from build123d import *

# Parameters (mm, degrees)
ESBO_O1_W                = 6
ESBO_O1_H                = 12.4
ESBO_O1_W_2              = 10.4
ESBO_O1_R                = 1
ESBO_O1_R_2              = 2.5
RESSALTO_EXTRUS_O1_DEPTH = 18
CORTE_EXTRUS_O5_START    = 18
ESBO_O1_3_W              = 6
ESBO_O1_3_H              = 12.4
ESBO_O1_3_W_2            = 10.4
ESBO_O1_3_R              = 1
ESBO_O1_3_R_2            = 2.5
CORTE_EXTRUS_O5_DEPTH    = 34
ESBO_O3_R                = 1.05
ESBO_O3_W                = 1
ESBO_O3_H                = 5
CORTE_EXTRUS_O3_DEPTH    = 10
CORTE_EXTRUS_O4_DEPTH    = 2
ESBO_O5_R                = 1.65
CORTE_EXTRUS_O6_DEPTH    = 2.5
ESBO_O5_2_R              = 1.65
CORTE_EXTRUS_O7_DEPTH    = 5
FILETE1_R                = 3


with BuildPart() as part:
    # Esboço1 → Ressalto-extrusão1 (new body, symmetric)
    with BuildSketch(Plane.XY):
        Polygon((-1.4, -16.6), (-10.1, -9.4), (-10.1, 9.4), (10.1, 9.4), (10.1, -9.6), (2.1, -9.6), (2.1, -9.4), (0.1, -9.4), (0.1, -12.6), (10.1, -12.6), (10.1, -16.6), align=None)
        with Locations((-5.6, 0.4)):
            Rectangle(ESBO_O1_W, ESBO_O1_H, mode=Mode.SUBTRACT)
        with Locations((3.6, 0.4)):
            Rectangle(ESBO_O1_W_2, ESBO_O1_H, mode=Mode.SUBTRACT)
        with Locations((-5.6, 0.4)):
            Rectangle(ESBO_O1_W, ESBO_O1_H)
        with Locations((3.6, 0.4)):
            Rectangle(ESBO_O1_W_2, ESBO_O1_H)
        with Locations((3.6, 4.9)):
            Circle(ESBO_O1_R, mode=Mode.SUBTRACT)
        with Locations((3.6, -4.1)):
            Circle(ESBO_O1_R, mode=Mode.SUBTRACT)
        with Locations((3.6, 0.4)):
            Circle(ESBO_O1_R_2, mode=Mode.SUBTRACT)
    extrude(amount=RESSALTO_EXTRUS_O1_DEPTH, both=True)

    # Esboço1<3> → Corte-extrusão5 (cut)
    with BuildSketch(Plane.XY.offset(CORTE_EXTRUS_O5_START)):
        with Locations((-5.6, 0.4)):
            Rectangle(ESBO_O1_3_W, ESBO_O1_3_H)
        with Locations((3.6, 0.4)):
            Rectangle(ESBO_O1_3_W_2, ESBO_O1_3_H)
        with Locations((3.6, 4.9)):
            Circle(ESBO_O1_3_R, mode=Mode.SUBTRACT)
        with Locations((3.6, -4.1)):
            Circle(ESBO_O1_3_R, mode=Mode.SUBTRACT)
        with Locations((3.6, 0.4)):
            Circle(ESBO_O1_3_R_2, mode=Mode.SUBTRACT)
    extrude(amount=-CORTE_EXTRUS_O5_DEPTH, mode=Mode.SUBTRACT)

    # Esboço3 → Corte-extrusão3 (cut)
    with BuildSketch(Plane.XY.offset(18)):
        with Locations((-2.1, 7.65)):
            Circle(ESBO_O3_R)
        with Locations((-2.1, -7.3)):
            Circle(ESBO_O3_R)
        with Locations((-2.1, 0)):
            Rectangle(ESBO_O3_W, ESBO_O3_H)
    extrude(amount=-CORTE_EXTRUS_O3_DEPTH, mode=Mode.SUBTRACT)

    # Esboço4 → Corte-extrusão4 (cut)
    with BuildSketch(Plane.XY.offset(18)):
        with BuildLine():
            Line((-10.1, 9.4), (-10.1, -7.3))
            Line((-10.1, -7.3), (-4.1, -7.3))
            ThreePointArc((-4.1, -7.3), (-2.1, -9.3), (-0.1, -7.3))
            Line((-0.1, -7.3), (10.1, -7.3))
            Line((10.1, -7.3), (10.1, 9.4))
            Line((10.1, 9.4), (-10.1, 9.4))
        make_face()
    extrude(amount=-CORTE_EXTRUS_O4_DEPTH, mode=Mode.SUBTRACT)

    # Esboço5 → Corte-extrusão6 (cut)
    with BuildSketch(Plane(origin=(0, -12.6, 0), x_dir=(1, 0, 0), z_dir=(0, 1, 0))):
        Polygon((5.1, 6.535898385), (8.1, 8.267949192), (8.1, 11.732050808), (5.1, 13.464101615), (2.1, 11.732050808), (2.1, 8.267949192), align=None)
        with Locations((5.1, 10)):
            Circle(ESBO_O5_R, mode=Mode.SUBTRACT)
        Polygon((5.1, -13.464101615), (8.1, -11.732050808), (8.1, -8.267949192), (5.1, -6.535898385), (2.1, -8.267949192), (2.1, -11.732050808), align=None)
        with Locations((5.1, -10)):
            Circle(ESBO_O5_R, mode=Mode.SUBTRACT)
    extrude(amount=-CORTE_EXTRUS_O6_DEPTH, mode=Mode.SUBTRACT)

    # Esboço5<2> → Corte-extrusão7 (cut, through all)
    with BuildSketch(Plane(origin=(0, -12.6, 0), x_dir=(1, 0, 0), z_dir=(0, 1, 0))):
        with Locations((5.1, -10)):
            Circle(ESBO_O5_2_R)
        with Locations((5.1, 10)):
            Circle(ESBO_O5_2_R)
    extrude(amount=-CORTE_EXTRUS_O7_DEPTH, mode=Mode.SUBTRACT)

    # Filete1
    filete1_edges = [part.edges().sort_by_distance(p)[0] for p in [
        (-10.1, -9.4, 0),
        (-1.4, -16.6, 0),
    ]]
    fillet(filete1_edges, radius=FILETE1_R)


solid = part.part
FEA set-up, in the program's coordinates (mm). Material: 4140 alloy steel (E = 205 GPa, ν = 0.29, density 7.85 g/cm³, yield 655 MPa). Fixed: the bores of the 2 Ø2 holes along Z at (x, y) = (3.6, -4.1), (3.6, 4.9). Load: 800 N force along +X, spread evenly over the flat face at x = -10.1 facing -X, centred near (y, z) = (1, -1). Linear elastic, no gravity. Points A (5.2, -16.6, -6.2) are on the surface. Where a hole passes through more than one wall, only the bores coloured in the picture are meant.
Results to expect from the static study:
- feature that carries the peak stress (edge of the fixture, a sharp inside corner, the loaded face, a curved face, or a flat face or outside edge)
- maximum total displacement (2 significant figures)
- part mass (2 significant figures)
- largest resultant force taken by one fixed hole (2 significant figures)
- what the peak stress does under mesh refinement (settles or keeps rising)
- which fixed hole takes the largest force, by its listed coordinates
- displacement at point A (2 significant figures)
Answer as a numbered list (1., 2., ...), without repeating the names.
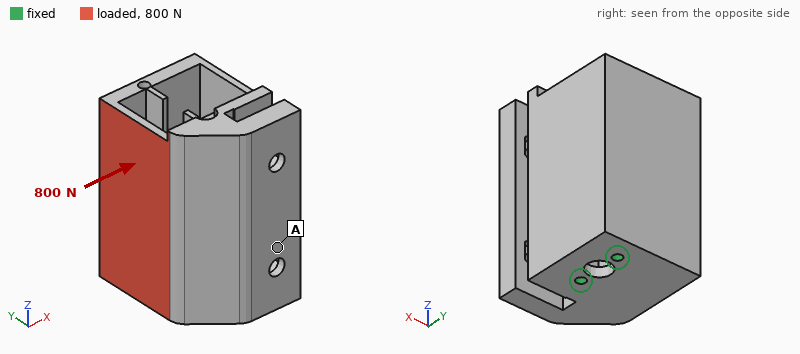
1. edge of the fixture
2. 0.21 mm
3. 72 g
4. 420 N
5. keeps rising
6. (3.6, 4.9)
7. 0.063 mm
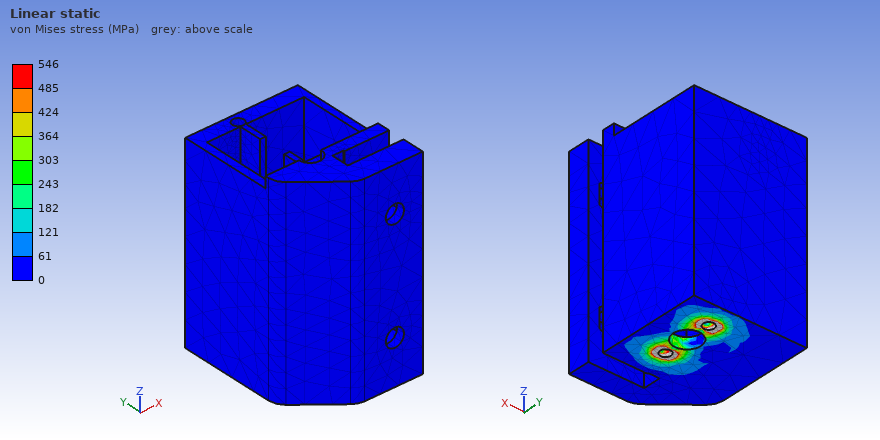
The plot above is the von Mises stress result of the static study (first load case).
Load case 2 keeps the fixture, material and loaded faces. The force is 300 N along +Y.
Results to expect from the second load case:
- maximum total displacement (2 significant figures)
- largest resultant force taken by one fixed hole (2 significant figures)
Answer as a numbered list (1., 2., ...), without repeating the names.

1. 20 µm
2. 560 N
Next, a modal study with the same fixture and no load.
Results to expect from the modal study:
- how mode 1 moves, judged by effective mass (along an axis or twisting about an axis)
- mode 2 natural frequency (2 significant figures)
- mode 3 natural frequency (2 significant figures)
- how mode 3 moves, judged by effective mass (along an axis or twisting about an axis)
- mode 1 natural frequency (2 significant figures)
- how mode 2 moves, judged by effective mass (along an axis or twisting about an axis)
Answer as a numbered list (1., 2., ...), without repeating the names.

1. along X
2. 3000 Hz
3. 8000 Hz
4. twisting about Z
5. 1400 Hz
6. along Y
